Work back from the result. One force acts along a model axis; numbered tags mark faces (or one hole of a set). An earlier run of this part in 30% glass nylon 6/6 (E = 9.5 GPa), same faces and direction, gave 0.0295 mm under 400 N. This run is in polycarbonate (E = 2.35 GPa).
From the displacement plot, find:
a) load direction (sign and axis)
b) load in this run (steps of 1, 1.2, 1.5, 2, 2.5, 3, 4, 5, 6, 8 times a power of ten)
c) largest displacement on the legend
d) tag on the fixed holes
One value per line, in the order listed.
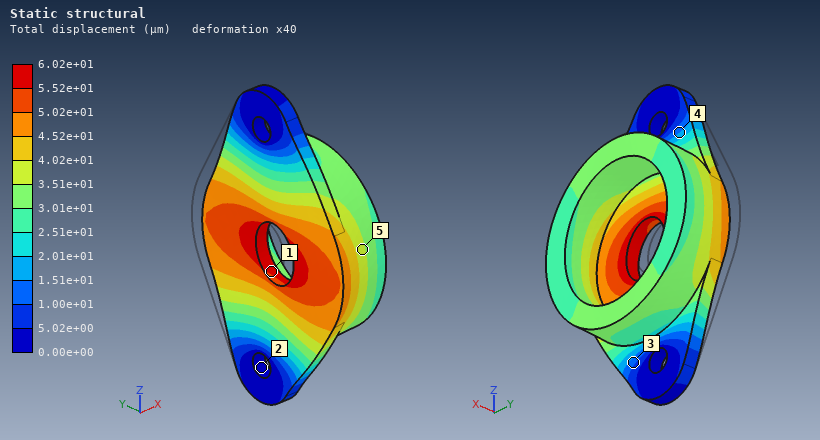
-Y
200 N
6.02e+01 µm
2
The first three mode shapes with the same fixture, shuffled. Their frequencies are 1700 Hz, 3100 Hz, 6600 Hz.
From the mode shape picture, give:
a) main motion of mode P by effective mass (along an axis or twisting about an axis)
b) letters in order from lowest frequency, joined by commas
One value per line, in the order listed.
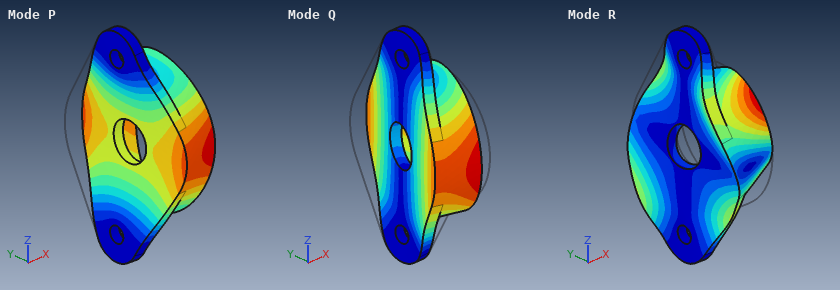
along X
Q, P, R
